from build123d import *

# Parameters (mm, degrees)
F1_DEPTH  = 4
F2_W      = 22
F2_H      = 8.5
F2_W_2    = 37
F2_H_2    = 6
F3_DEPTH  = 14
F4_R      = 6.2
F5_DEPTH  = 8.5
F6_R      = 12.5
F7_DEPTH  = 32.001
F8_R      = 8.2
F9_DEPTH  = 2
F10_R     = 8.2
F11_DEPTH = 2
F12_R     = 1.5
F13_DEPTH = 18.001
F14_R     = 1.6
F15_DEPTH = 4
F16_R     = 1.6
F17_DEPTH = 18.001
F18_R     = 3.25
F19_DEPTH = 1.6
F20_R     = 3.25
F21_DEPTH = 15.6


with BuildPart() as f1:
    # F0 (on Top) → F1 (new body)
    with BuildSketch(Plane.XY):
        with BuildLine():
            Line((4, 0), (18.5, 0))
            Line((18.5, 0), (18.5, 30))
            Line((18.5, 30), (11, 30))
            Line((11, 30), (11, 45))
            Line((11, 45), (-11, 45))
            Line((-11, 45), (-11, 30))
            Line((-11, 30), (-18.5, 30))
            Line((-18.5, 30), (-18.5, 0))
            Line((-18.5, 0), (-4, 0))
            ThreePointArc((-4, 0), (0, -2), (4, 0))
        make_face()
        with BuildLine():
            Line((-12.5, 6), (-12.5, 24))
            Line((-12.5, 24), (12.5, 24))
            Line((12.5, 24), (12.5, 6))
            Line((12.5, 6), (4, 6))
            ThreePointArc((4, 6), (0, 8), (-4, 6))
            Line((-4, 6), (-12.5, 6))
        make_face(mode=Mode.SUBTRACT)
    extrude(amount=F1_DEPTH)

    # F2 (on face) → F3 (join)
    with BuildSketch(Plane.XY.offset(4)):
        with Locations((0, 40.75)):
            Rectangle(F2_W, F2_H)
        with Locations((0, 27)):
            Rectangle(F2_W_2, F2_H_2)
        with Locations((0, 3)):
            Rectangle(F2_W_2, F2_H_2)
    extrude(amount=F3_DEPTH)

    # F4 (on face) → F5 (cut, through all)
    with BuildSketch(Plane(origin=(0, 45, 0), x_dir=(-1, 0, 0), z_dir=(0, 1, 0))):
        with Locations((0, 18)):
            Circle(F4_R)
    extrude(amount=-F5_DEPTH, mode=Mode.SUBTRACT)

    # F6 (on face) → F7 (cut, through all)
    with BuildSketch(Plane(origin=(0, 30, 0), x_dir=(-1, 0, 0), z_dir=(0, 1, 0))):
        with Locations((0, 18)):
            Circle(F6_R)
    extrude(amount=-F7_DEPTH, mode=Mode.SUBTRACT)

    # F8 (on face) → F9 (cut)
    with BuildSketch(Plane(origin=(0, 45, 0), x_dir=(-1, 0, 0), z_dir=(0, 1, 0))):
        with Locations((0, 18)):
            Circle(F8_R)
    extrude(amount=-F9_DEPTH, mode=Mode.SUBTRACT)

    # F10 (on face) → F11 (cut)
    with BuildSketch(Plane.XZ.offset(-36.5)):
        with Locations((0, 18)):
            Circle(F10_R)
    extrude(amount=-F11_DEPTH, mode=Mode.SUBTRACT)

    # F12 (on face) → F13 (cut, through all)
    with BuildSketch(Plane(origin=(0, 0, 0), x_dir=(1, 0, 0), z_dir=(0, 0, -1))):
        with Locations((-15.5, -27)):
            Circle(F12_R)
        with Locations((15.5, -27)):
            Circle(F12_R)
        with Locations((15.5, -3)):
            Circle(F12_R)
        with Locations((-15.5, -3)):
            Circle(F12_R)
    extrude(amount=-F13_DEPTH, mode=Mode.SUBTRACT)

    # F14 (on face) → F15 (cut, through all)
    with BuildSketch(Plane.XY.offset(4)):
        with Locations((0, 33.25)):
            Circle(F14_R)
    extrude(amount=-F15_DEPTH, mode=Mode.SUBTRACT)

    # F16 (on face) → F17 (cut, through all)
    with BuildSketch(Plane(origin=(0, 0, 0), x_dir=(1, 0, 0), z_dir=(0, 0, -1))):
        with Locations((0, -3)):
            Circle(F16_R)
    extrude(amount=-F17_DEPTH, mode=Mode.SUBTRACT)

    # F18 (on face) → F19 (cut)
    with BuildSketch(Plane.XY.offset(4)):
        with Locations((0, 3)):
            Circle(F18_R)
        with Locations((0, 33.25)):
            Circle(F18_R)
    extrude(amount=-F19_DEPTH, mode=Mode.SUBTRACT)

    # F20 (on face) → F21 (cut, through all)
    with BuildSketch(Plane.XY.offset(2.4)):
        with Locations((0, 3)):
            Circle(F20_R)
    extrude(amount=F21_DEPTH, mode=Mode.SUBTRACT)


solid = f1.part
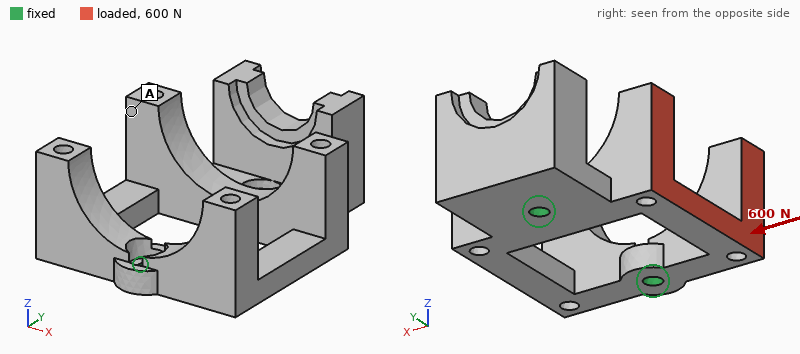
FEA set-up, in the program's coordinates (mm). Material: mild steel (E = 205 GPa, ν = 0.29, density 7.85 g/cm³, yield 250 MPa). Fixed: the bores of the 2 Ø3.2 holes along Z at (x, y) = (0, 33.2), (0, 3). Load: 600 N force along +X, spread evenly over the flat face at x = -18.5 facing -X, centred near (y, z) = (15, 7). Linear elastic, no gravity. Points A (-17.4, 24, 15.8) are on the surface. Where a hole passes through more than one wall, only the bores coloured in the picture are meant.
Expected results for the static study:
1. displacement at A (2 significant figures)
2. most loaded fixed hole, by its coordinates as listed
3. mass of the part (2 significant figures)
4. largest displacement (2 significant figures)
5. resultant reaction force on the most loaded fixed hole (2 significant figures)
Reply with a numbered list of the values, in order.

1. 24 µm
2. (0, 3)
3. 67 g
4. 38 µm
5. 330 N
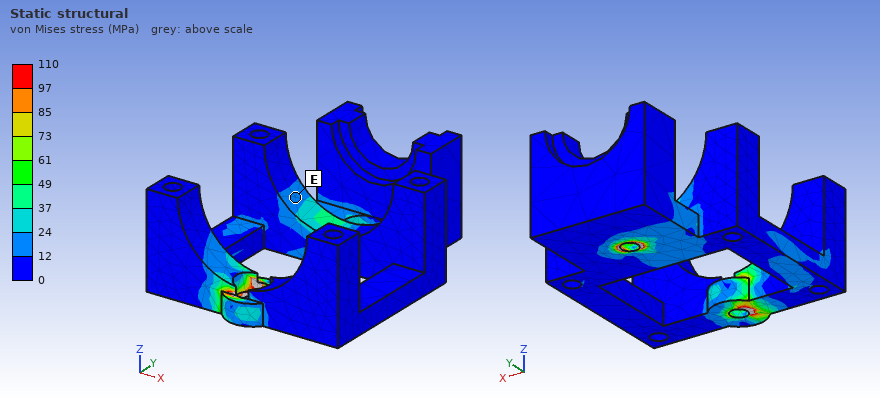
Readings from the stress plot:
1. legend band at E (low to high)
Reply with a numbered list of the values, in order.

1. 12 to 24 MPa
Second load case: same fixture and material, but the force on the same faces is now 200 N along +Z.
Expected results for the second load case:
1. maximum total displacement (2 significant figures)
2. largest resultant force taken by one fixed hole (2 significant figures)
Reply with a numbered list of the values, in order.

1. 37 µm
2. 100 N
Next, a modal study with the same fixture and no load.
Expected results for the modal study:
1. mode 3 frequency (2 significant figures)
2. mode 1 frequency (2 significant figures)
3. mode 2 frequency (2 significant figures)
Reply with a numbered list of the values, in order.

1. 5700 Hz
2. 3400 Hz
3. 4300 Hz
